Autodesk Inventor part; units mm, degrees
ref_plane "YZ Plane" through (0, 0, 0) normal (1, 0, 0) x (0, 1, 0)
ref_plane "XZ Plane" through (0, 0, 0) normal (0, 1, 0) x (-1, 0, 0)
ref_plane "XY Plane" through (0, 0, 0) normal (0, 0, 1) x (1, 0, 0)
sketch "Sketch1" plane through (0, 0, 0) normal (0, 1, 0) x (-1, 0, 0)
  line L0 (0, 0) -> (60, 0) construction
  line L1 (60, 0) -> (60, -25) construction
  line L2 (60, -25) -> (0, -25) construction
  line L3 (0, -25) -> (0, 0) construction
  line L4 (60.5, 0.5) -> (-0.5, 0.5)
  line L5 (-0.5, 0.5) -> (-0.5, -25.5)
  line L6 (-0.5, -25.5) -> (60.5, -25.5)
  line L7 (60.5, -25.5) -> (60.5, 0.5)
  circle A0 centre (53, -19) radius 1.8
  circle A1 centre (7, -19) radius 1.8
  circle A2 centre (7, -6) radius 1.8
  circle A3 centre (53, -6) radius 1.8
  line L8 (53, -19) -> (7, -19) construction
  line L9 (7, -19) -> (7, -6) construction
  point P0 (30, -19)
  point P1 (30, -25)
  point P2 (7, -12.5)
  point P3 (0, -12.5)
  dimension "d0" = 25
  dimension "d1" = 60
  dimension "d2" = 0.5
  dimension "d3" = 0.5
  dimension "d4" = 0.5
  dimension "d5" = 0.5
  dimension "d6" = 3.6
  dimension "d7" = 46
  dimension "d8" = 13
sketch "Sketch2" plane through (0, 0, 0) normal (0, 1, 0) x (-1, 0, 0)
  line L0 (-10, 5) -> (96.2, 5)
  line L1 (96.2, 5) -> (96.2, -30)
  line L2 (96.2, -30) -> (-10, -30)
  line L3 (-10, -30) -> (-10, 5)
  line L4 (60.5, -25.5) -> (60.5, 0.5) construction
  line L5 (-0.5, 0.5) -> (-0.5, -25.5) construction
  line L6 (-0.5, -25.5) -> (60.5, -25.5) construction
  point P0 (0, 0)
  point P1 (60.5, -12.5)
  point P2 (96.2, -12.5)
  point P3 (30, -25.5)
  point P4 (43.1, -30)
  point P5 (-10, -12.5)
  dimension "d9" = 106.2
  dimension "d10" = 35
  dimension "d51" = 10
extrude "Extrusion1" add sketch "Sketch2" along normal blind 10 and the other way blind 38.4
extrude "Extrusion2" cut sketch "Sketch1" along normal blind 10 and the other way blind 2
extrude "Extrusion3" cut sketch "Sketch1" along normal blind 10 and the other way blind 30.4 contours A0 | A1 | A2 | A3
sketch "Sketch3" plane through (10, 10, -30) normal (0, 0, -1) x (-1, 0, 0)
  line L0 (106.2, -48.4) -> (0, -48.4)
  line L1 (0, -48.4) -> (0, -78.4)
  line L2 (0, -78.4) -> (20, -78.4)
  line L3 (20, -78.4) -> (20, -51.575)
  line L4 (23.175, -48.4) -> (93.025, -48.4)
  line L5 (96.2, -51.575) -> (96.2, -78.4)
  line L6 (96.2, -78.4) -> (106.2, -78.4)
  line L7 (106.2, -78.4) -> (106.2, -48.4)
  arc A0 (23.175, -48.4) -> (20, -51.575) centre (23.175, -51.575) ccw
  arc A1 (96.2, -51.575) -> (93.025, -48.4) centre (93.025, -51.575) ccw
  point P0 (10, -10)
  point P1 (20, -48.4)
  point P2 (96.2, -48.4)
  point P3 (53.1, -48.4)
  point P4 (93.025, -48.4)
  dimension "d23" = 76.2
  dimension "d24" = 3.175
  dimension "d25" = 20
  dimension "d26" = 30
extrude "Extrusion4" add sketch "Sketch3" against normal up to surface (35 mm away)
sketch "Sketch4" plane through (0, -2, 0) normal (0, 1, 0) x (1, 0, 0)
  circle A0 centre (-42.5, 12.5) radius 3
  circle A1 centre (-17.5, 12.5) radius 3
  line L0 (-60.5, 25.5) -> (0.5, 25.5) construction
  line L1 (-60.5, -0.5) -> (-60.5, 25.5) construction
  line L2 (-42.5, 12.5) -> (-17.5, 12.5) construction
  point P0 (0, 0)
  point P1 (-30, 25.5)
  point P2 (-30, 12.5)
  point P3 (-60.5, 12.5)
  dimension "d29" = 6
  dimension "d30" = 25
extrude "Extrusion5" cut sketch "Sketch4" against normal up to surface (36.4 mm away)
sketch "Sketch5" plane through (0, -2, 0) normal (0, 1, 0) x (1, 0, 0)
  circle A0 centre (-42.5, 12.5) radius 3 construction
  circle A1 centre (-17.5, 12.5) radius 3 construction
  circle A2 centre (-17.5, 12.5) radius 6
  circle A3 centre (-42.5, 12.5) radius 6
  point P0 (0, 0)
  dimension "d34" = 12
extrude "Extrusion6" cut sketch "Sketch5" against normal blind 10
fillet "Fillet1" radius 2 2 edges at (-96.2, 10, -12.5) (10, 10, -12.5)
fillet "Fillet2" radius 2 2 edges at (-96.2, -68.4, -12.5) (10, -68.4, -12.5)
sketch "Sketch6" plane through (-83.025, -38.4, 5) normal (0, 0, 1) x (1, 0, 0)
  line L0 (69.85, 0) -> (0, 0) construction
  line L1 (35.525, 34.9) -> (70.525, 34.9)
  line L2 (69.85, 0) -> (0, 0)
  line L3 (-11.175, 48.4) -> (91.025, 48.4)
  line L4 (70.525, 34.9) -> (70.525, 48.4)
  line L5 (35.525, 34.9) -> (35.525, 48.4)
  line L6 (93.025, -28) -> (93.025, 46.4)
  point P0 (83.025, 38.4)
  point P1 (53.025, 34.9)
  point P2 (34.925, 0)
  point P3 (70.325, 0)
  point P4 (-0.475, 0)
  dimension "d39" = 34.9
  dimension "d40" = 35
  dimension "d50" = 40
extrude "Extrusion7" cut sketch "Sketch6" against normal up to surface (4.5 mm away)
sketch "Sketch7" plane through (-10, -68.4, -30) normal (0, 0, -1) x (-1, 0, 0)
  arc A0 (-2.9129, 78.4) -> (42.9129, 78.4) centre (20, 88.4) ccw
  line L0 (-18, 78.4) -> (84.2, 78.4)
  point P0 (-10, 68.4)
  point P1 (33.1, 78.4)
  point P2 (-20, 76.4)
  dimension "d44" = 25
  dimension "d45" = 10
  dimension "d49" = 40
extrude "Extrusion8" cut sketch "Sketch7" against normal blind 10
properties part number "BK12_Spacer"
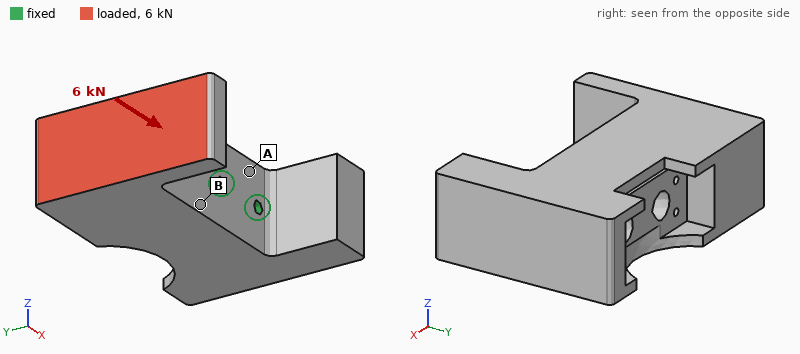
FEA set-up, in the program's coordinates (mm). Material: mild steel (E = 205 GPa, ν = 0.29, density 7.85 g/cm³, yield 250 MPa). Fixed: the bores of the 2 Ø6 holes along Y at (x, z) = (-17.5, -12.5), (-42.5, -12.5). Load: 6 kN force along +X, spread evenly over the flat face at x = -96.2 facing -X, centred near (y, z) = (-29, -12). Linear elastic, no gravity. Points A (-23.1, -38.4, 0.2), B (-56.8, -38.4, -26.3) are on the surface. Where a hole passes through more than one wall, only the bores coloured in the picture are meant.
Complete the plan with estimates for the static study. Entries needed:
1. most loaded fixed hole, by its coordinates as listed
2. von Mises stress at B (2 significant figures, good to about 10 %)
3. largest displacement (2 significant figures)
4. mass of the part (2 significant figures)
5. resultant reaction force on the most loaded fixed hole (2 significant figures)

(-42.5, -12.5)
9.8 MPa
27 µm
1.4 kg
4.7 kN
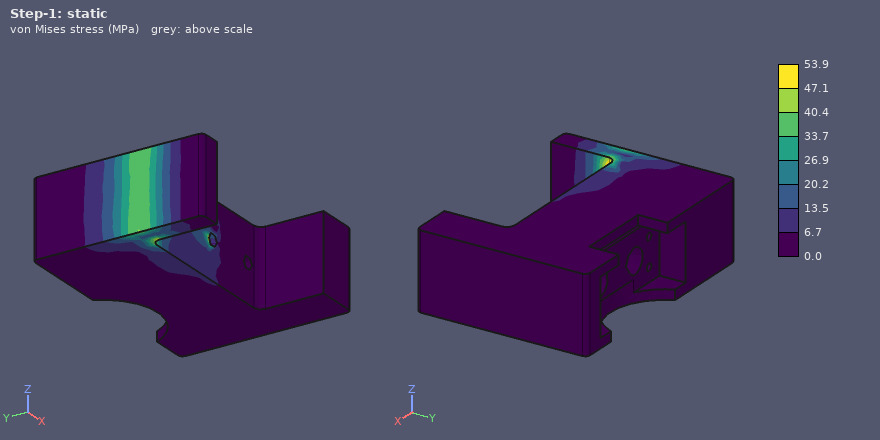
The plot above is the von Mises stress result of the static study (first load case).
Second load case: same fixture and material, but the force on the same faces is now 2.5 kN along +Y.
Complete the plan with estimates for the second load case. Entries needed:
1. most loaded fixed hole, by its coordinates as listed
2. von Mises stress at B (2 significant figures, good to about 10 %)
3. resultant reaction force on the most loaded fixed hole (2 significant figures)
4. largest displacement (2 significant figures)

(-42.5, -12.5)
12 MPa
4.3 kN
16 µm
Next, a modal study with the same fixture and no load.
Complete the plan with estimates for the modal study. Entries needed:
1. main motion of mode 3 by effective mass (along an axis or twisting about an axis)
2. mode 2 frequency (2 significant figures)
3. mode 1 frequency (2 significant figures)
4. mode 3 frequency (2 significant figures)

twisting about X
4200 Hz
4100 Hz
5800 Hz
